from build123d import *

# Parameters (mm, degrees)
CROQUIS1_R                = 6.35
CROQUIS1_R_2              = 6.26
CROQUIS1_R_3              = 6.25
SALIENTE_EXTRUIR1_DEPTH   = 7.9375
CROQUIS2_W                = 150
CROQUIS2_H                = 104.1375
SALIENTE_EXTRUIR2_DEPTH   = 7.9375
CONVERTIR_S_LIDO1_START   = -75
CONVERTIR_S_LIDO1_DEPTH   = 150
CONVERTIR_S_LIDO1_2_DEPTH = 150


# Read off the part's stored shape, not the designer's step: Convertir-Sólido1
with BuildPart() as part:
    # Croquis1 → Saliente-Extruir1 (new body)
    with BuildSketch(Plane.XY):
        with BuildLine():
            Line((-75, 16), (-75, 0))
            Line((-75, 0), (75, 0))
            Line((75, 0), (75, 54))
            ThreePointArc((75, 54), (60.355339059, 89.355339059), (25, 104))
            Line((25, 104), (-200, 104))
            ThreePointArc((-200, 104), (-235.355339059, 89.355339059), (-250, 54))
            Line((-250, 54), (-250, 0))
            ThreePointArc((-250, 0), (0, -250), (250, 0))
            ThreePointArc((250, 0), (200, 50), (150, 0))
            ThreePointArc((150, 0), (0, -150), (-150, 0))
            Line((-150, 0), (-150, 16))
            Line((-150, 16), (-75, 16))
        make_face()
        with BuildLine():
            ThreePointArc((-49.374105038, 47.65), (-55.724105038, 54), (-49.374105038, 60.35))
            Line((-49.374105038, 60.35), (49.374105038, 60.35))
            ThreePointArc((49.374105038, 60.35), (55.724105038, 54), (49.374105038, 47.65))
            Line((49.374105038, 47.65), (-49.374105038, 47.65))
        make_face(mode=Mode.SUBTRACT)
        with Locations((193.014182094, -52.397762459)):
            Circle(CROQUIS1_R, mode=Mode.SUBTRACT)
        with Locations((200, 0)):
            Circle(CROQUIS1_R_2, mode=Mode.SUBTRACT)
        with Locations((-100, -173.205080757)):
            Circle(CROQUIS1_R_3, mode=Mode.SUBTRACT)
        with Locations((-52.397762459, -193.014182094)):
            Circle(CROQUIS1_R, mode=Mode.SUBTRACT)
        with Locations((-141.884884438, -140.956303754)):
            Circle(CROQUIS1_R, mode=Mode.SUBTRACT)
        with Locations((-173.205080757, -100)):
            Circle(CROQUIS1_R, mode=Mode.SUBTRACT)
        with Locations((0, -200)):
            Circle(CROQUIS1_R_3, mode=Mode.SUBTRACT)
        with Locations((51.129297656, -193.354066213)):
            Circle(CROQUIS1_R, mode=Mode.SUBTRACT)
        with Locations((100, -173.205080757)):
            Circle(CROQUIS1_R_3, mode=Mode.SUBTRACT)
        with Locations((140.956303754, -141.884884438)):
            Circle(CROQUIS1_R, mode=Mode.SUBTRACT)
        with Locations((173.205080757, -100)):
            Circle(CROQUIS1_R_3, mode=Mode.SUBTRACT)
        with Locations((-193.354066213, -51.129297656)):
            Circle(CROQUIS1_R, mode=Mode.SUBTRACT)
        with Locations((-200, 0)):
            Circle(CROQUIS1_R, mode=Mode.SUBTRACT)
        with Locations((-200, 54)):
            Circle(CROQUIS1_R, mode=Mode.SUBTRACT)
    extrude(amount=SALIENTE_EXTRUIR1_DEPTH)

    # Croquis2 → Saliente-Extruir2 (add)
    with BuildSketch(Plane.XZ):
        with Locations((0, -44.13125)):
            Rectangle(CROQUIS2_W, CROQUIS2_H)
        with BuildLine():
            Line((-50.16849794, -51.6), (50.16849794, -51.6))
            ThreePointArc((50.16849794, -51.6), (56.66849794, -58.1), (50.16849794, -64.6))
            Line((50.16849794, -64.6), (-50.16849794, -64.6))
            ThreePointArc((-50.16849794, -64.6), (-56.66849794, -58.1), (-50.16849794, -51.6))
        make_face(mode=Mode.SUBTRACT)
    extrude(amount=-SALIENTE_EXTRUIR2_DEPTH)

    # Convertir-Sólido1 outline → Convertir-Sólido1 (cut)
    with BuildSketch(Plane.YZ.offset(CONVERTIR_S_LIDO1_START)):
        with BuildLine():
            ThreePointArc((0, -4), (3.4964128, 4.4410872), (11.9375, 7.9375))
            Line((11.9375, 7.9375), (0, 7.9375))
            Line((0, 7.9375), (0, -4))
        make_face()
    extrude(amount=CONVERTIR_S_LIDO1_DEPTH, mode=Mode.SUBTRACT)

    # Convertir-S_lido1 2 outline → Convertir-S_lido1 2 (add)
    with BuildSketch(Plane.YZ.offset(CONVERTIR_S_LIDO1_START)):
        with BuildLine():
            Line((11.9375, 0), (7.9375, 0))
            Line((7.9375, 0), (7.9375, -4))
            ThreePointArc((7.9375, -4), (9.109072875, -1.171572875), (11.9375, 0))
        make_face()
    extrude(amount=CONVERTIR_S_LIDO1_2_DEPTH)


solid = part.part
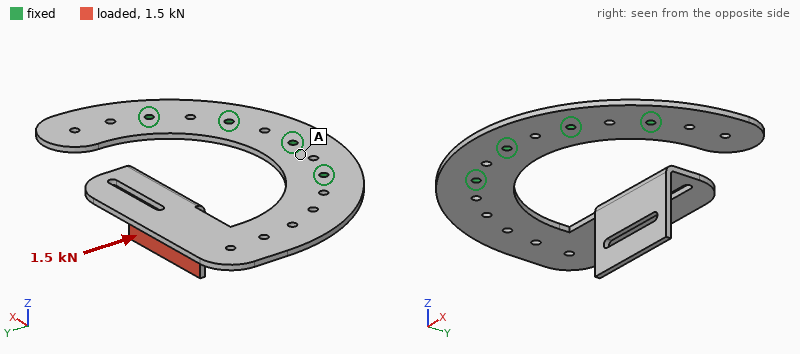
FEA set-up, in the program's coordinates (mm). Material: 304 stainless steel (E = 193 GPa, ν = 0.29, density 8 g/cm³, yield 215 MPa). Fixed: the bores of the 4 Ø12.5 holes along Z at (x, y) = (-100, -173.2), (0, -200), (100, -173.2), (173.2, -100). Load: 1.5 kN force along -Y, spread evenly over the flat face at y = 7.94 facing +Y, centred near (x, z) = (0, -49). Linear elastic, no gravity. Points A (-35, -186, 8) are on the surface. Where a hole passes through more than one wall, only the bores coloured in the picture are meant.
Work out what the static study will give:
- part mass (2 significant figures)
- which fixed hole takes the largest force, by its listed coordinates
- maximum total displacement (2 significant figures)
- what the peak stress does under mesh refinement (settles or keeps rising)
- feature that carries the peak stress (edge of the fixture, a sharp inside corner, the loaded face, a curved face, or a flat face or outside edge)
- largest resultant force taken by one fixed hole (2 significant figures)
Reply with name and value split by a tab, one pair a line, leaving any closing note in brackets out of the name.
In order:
part mass	6.8 kg
which fixed hole takes the largest force, by its listed coordinates	(0, -200)
maximum total displacement	4.5 mm
what the peak stress does under mesh refinement	keeps rising
feature that carries the peak stress	a sharp inside corner
largest resultant force taken by one fixed hole	1.1 kN
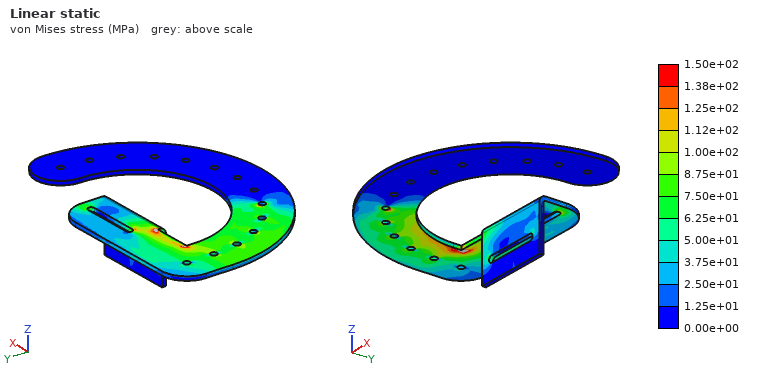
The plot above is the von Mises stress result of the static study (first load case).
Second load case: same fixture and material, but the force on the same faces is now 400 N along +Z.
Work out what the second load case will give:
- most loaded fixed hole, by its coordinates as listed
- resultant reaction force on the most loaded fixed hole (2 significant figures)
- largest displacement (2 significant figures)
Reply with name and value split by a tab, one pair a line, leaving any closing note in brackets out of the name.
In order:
most loaded fixed hole, by its coordinates as listed	(-100, -173.2)
resultant reaction force on the most loaded fixed hole	390 N
largest displacement	6.3 mm
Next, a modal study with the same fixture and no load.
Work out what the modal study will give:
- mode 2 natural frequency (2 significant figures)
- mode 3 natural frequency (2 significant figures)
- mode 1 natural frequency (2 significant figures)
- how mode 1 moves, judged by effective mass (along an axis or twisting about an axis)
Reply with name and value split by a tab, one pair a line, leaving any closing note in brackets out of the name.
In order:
mode 2 natural frequency	58 Hz
mode 3 natural frequency	150 Hz
mode 1 natural frequency	33 Hz
how mode 1 moves, judged by effective mass	along Z
